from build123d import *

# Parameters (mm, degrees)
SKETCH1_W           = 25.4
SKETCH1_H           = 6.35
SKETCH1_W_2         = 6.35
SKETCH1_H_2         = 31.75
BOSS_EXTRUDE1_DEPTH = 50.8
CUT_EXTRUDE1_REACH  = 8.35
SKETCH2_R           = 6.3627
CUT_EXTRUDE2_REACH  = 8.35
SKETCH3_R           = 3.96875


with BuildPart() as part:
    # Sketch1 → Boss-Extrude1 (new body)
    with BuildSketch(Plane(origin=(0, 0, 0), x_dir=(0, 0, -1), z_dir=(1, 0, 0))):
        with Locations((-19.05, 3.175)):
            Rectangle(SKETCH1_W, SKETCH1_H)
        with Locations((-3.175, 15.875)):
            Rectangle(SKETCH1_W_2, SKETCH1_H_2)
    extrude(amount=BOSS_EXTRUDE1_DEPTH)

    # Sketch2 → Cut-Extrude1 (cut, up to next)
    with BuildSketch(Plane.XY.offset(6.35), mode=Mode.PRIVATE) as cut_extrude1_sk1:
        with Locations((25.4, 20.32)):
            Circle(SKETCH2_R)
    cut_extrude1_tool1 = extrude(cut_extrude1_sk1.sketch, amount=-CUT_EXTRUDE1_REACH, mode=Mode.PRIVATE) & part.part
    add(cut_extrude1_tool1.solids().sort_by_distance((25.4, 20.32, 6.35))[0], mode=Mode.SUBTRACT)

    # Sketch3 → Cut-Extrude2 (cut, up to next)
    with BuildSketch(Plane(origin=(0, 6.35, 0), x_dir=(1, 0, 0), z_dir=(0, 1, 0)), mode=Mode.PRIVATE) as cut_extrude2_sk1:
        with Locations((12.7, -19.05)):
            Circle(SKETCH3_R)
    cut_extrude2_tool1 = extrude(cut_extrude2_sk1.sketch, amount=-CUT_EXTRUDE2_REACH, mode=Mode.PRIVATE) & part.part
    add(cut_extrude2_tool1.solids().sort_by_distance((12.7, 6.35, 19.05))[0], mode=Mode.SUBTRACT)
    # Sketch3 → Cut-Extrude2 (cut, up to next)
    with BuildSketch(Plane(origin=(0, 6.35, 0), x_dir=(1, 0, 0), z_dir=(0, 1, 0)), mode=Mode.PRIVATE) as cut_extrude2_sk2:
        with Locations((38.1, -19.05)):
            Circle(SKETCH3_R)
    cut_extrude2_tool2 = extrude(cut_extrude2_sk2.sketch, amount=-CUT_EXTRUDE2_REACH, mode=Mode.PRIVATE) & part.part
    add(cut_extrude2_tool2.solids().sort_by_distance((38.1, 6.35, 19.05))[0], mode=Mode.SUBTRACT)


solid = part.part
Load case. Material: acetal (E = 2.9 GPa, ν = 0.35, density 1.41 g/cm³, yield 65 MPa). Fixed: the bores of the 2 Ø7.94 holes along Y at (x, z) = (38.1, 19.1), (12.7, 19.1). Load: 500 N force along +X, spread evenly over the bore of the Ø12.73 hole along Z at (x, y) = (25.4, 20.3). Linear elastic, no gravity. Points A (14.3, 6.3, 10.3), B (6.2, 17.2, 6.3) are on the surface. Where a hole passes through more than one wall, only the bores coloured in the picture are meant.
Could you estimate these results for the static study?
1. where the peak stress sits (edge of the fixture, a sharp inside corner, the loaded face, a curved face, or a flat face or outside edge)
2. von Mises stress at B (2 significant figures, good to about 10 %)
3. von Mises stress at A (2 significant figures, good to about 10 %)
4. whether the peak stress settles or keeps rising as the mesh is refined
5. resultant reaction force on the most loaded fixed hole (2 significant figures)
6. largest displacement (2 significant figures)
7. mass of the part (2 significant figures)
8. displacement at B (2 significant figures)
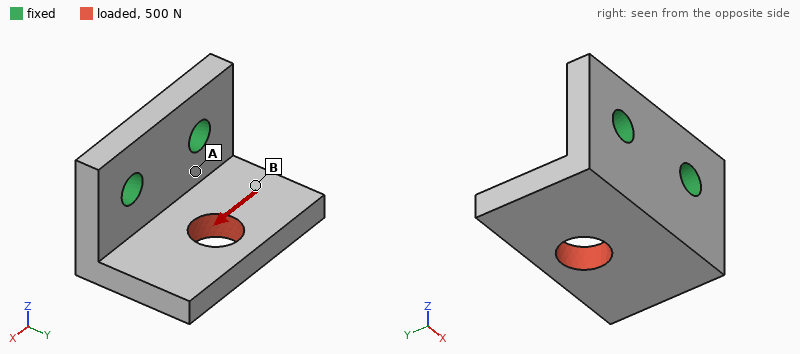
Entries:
edge of the fixture
4.5 MPa
10 MPa
keeps rising
420 N
0.38 mm
24 g
0.22 mm
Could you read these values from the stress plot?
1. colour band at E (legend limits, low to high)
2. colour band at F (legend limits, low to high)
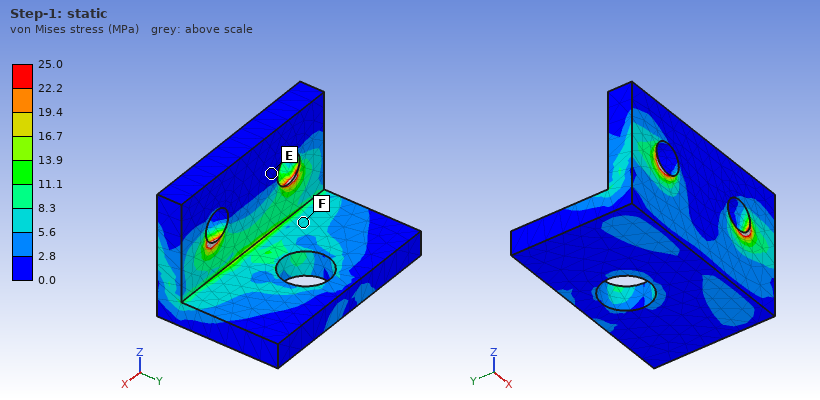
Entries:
0.0 to 2.8 MPa
5.6 to 8.3 MPa
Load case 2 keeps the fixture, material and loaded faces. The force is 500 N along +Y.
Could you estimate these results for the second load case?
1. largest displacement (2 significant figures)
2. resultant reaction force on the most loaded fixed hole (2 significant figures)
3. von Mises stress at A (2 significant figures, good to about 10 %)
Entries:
0.52 mm
250 N
12 MPa
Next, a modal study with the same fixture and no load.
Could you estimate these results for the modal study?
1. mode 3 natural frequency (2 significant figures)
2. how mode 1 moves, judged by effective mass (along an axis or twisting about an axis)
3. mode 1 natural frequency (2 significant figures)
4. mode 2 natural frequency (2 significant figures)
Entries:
2600 Hz
along Z
1100 Hz
1800 Hz
